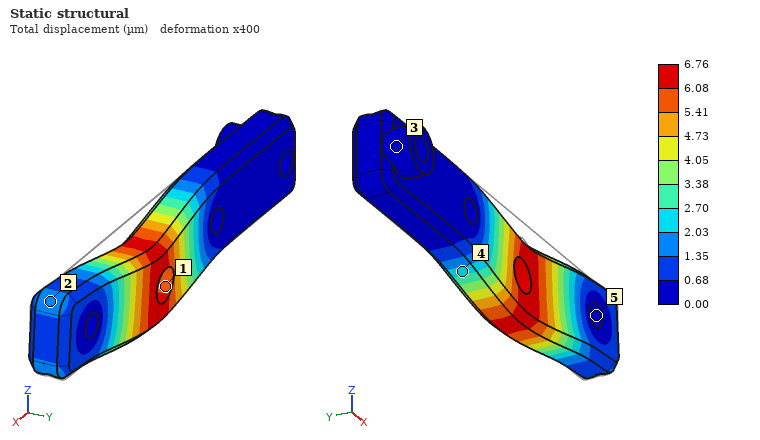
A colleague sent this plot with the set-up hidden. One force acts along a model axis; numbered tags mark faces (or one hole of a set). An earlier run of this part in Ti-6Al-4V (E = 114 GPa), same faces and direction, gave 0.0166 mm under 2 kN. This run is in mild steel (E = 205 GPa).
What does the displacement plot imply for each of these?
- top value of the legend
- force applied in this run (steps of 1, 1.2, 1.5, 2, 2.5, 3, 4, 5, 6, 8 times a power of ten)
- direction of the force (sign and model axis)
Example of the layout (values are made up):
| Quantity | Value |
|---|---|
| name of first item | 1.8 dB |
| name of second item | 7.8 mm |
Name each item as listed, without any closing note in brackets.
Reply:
| Quantity | Value |
|---|---|
| top value of the legend | 6.76 µm |
| force applied in this run | 1.5 kN |
| direction of the force | -Z |
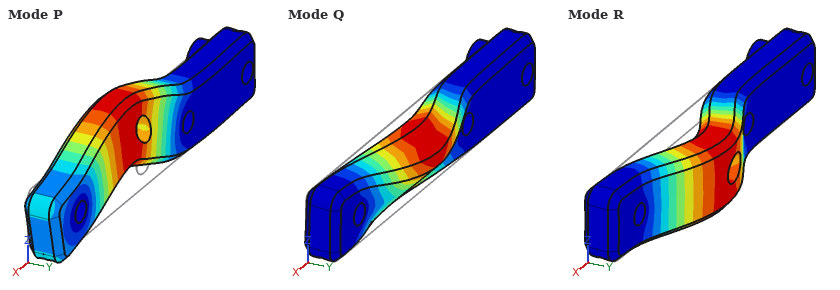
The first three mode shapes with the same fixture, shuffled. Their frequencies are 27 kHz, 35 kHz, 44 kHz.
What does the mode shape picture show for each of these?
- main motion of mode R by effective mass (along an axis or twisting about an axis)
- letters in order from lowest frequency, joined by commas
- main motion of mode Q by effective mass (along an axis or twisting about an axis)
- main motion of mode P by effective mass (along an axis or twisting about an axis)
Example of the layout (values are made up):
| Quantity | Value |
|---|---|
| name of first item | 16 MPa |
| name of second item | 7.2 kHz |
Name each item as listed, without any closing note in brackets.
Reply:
| Quantity | Value |
|---|---|
| main motion of mode R by effective mass | along Y |
| letters in order from lowest frequency, joined by commas | R, P, Q |
| main motion of mode Q by effective mass | twisting about X |
| main motion of mode P by effective mass | along Z |
